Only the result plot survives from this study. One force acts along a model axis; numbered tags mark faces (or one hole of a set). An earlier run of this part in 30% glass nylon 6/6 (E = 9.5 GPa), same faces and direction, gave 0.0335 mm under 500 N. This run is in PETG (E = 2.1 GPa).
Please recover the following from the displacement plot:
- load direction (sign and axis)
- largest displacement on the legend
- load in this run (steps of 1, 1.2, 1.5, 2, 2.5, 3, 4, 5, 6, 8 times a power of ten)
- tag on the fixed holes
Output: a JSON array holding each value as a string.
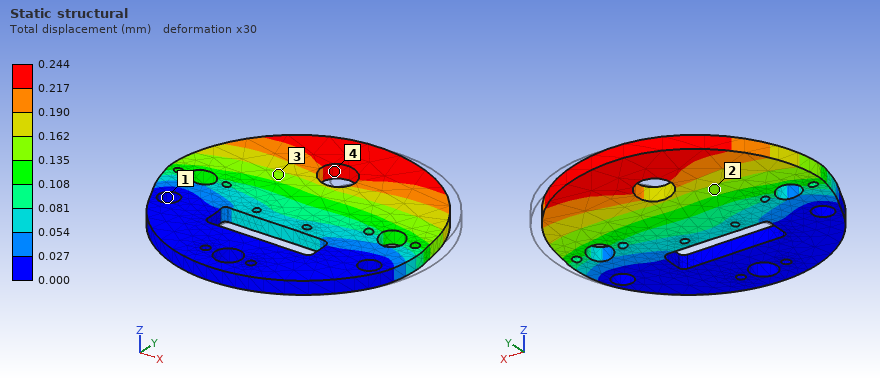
["-X", "0.244 mm", "800 N", "1"]
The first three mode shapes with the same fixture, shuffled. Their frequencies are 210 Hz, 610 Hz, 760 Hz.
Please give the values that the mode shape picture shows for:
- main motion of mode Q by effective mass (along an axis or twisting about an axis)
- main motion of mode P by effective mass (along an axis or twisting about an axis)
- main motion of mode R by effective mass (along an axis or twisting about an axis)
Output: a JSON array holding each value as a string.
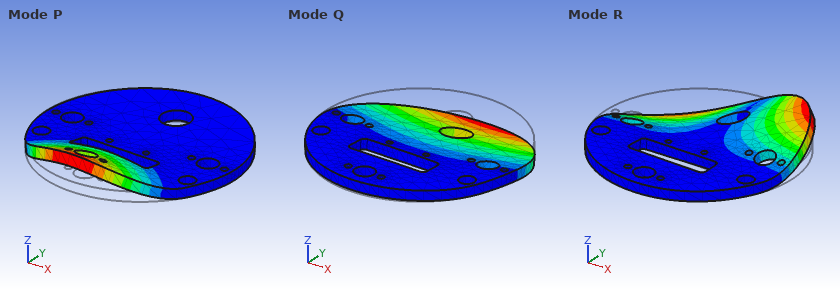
["along Z", "along Z", "twisting about Y"]
